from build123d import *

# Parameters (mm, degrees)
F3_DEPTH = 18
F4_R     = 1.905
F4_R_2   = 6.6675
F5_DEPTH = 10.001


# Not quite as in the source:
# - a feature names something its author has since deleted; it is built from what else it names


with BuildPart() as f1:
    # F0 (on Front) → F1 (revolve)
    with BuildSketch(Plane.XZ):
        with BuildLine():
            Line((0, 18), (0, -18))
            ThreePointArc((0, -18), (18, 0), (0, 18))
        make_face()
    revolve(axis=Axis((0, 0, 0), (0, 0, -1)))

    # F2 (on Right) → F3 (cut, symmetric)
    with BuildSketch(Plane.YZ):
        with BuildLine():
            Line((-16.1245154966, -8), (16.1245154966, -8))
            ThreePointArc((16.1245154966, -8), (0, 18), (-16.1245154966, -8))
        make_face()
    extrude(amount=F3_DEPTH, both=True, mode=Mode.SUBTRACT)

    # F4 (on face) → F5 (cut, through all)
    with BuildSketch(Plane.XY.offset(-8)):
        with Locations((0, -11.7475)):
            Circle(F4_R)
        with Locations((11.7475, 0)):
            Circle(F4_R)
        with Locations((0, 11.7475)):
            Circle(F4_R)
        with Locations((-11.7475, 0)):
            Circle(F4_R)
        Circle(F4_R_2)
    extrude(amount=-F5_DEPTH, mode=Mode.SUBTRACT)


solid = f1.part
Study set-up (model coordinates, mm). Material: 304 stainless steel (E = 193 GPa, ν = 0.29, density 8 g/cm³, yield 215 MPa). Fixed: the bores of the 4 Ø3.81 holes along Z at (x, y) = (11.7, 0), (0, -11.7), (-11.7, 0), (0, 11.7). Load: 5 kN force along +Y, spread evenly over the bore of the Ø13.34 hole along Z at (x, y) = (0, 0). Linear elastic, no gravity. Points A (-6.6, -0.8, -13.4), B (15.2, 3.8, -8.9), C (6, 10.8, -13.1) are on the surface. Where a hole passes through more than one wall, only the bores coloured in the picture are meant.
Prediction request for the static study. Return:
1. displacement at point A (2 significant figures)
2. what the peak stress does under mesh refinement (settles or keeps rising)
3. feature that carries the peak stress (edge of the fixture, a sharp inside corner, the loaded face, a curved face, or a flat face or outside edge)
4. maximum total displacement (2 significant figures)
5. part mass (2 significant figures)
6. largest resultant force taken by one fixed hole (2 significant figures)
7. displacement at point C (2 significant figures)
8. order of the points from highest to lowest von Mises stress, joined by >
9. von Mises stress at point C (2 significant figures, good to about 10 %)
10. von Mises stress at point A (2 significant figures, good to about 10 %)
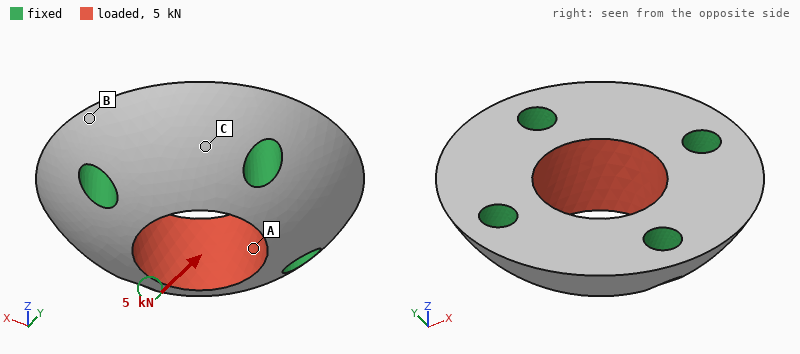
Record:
1.1 µm
keeps rising
edge of the fixture
1.9 µm
24 g
1.3 kN
0.77 µm
A > C > B
15 MPa
31 MPa
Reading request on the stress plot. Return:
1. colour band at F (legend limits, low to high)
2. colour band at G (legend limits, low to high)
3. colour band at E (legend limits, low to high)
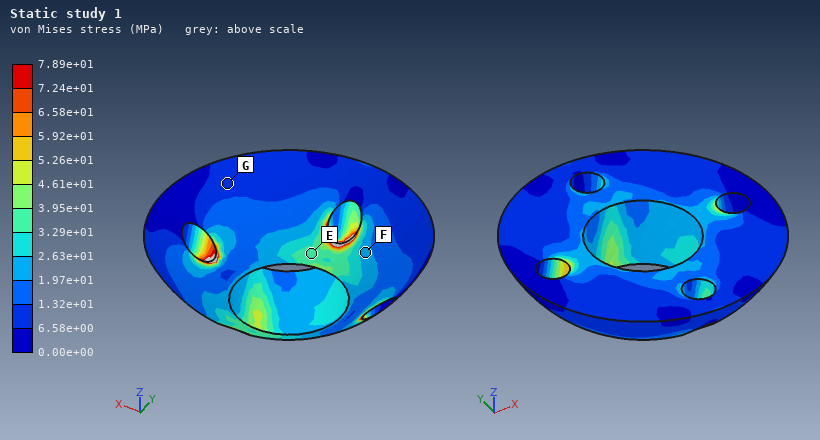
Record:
1.97e+01 to 2.63e+01 MPa
6.58e+00 to 1.32e+01 MPa
3.29e+01 to 3.95e+01 MPa
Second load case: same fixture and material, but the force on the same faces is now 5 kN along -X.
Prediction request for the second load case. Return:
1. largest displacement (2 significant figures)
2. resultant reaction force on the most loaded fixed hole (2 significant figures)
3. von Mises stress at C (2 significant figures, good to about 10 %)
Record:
1.9 µm
1.3 kN
17 MPa
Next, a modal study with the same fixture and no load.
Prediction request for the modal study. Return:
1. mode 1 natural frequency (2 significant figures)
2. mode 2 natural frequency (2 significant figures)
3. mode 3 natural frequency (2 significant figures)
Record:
63 kHz
66 kHz
66 kHz
